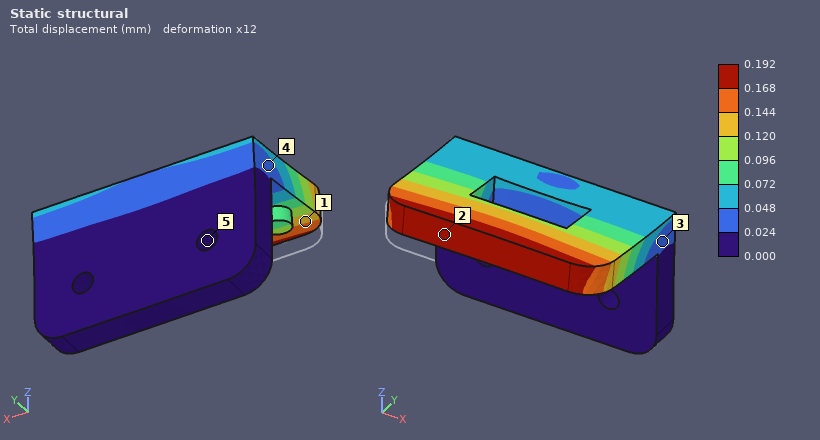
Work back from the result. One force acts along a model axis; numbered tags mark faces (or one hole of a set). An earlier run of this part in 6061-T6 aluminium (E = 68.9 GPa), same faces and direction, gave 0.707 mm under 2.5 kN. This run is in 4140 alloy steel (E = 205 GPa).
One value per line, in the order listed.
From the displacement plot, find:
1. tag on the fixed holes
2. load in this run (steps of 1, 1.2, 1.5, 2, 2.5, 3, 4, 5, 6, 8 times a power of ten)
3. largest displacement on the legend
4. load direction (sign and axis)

5
2 kN
0.192 mm
+Z
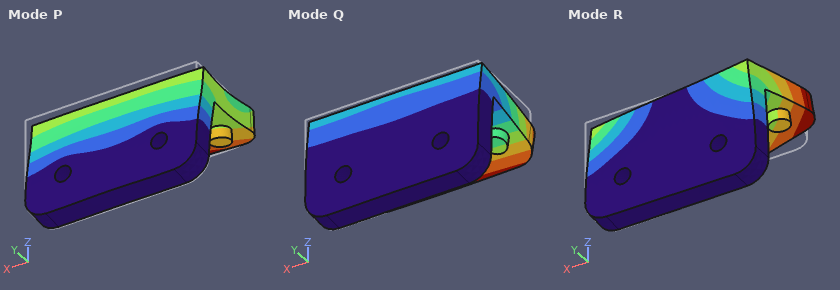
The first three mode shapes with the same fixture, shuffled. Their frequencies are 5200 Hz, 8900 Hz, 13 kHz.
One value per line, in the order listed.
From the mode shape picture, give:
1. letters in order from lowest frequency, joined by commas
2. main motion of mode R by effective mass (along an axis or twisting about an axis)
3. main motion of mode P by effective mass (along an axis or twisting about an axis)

Q, R, P
along X
along Y
